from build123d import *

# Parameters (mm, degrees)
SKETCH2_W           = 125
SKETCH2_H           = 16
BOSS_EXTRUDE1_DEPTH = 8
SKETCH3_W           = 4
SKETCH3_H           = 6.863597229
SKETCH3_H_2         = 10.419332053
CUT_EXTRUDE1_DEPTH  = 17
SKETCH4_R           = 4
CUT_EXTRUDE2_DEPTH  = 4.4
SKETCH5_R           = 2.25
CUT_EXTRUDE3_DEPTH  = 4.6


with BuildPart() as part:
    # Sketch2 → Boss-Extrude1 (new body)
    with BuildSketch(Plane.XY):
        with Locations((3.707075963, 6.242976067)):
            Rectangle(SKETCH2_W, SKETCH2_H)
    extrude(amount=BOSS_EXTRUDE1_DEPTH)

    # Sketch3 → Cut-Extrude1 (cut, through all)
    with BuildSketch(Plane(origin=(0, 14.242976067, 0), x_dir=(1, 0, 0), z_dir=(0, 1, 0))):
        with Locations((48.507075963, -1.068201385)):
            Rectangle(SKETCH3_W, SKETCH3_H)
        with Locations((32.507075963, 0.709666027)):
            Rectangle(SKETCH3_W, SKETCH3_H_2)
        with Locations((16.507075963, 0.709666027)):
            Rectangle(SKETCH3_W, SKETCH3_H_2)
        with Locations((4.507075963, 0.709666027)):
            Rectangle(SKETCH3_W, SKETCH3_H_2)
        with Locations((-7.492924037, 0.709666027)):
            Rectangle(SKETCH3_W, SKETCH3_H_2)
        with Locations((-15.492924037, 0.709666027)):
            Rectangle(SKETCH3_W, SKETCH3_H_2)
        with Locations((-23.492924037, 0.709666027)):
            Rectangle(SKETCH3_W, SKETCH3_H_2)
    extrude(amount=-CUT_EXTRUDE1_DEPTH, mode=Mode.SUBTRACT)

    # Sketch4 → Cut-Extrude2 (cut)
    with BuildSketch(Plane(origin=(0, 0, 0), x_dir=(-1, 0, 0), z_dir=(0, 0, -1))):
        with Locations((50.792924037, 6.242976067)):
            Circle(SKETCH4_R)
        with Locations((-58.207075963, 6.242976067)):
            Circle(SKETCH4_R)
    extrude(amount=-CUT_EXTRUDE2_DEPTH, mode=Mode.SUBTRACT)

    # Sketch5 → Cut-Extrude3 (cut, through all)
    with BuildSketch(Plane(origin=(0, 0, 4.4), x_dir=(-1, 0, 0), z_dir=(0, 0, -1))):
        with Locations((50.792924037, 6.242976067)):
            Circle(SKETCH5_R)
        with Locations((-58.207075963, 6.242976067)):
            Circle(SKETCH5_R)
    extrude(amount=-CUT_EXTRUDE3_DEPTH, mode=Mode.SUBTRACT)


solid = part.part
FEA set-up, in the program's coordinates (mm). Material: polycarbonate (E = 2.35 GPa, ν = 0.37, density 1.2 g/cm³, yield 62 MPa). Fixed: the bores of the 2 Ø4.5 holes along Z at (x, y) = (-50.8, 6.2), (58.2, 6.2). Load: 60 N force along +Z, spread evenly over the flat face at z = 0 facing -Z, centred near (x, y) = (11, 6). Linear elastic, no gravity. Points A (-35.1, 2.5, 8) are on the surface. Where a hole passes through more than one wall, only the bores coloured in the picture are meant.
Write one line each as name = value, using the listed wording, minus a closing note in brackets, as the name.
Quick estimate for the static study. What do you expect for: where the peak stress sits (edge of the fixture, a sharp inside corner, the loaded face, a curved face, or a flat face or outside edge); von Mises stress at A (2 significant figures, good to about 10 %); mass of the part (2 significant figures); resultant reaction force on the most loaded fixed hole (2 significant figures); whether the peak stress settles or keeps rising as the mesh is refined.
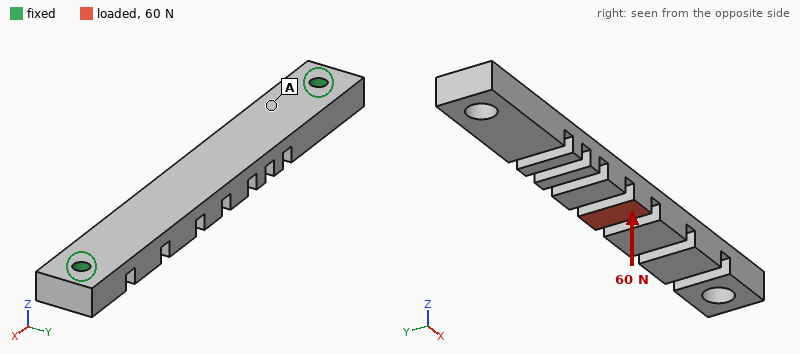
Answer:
where the peak stress sits = edge of the fixture
von Mises stress at A = 3.2 MPa
mass of the part = 16 g
resultant reaction force on the most loaded fixed hole = 35 N
whether the peak stress settles or keeps rising as the mesh is refined = keeps rising
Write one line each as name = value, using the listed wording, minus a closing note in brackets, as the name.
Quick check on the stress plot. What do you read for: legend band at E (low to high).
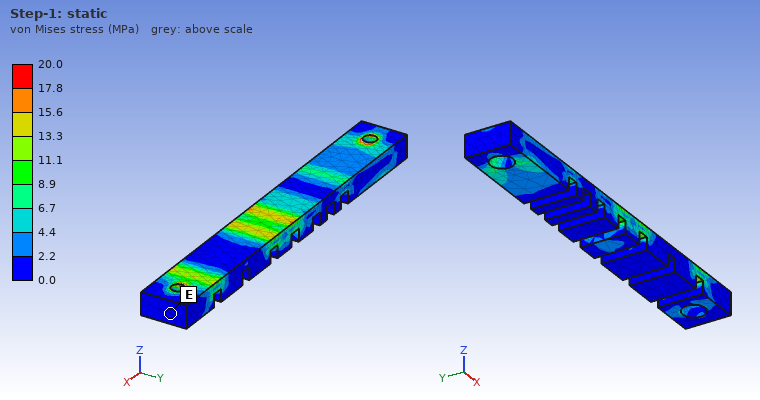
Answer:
legend band at E = 0.0 to 2.2 MPa
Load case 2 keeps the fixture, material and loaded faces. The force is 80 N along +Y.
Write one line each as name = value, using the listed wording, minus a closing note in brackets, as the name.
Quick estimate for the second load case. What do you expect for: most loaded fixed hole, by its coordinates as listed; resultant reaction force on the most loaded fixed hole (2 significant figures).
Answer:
most loaded fixed hole, by its coordinates as listed = (58.2, 6.2)
resultant reaction force on the most loaded fixed hole = 45 N
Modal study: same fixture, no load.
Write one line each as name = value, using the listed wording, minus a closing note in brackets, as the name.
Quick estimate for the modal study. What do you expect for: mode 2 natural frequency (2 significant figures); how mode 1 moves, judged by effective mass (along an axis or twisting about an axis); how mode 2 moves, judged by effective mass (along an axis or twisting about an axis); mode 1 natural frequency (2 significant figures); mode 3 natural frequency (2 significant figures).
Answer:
mode 2 natural frequency = 1100 Hz
how mode 1 moves, judged by effective mass = along Z
how mode 2 moves, judged by effective mass = along Y
mode 1 natural frequency = 500 Hz
mode 3 natural frequency = 1200 Hz
